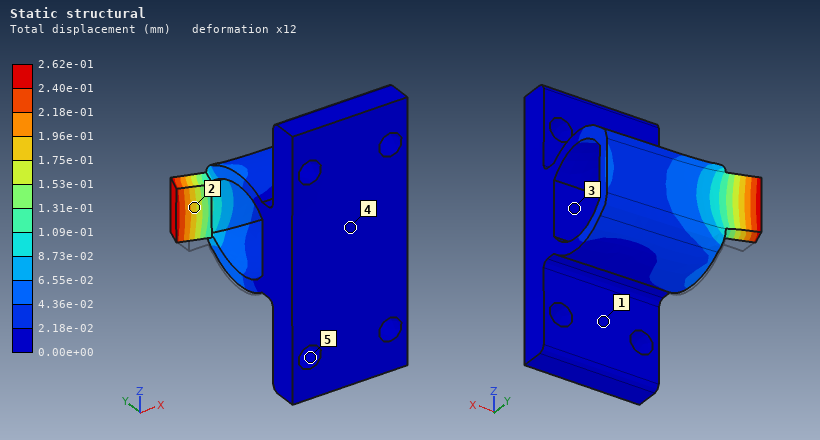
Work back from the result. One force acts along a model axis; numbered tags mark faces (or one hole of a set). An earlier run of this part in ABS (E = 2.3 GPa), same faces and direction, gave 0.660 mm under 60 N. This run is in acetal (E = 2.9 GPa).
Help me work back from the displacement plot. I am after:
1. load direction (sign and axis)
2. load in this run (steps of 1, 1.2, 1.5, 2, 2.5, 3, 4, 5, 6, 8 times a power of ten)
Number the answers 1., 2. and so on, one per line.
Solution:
1. +Y
2. 30 N
